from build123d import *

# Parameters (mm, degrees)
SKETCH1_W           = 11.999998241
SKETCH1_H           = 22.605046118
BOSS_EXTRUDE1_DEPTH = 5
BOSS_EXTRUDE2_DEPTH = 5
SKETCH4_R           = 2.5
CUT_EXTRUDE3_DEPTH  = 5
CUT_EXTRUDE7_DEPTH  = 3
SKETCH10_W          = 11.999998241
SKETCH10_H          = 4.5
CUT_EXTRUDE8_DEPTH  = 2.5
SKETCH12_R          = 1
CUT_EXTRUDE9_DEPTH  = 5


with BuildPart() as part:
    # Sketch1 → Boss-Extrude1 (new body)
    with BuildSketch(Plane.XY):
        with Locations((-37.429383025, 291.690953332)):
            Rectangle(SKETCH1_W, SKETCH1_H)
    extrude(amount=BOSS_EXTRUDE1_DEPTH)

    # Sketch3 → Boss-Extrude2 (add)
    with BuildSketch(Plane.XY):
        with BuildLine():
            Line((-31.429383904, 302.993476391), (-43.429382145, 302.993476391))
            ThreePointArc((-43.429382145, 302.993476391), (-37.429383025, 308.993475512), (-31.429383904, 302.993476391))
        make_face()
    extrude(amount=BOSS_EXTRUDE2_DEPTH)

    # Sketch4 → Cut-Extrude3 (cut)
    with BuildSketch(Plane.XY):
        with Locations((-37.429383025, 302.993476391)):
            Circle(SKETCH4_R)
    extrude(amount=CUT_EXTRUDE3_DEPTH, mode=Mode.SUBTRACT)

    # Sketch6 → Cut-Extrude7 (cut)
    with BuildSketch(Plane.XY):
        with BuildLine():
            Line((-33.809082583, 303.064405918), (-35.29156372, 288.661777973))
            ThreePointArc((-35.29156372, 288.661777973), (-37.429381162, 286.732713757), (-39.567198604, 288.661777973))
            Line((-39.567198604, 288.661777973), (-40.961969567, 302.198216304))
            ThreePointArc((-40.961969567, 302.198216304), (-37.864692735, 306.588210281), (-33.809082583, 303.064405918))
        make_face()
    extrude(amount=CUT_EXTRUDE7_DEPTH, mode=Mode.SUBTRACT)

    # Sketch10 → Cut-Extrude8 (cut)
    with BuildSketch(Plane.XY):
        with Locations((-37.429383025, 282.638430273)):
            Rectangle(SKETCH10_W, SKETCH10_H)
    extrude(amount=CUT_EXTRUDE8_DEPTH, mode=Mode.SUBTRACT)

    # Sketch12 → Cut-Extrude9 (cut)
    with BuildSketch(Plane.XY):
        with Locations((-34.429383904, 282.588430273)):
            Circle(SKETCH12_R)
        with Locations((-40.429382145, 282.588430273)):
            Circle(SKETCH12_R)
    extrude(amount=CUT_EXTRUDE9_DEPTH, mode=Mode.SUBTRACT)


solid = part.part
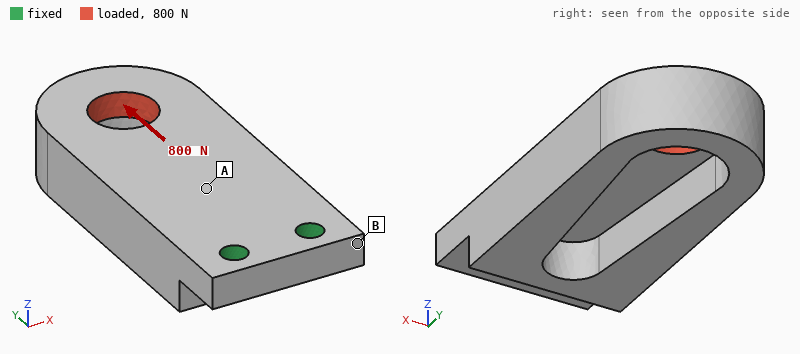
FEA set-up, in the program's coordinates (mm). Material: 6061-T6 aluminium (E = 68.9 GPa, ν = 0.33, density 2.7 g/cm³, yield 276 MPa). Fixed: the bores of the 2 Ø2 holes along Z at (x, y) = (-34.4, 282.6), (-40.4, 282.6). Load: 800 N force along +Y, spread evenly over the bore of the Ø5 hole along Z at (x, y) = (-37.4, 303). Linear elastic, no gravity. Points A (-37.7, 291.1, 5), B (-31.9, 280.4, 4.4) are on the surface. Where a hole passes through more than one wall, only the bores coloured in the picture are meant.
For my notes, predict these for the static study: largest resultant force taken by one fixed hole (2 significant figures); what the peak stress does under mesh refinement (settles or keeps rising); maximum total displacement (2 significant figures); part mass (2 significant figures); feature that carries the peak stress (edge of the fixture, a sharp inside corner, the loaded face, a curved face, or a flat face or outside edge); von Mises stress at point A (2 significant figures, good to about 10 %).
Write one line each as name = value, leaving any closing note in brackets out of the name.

largest resultant force taken by one fixed hole = 400 N
what the peak stress does under mesh refinement = keeps rising
maximum total displacement = 54 µm
part mass = 3.0 g
feature that carries the peak stress = edge of the fixture
von Mises stress at point A = 39 MPa
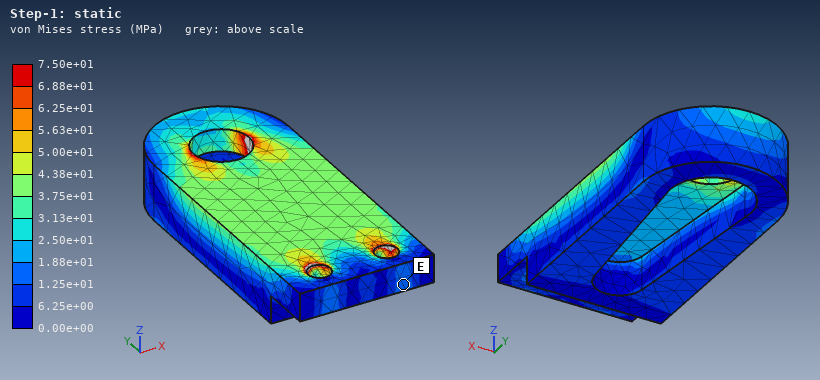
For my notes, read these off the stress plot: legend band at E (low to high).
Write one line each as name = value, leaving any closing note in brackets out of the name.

legend band at E = 1.25e+01 to 1.88e+01 MPa
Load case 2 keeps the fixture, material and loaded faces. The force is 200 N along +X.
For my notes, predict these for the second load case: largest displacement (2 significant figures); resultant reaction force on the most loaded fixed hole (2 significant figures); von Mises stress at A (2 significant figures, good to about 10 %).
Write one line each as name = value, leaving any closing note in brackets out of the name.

largest displacement = 40 µm
resultant reaction force on the most loaded fixed hole = 550 N
von Mises stress at A = 23 MPa
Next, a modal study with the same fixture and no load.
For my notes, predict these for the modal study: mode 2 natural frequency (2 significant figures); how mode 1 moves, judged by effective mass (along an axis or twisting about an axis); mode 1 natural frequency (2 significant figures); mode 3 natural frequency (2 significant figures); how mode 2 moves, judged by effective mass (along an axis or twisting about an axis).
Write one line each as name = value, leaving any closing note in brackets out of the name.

mode 2 natural frequency = 11 kHz
how mode 1 moves, judged by effective mass = along Z
mode 1 natural frequency = 3900 Hz
mode 3 natural frequency = 14 kHz
how mode 2 moves, judged by effective mass = along X
